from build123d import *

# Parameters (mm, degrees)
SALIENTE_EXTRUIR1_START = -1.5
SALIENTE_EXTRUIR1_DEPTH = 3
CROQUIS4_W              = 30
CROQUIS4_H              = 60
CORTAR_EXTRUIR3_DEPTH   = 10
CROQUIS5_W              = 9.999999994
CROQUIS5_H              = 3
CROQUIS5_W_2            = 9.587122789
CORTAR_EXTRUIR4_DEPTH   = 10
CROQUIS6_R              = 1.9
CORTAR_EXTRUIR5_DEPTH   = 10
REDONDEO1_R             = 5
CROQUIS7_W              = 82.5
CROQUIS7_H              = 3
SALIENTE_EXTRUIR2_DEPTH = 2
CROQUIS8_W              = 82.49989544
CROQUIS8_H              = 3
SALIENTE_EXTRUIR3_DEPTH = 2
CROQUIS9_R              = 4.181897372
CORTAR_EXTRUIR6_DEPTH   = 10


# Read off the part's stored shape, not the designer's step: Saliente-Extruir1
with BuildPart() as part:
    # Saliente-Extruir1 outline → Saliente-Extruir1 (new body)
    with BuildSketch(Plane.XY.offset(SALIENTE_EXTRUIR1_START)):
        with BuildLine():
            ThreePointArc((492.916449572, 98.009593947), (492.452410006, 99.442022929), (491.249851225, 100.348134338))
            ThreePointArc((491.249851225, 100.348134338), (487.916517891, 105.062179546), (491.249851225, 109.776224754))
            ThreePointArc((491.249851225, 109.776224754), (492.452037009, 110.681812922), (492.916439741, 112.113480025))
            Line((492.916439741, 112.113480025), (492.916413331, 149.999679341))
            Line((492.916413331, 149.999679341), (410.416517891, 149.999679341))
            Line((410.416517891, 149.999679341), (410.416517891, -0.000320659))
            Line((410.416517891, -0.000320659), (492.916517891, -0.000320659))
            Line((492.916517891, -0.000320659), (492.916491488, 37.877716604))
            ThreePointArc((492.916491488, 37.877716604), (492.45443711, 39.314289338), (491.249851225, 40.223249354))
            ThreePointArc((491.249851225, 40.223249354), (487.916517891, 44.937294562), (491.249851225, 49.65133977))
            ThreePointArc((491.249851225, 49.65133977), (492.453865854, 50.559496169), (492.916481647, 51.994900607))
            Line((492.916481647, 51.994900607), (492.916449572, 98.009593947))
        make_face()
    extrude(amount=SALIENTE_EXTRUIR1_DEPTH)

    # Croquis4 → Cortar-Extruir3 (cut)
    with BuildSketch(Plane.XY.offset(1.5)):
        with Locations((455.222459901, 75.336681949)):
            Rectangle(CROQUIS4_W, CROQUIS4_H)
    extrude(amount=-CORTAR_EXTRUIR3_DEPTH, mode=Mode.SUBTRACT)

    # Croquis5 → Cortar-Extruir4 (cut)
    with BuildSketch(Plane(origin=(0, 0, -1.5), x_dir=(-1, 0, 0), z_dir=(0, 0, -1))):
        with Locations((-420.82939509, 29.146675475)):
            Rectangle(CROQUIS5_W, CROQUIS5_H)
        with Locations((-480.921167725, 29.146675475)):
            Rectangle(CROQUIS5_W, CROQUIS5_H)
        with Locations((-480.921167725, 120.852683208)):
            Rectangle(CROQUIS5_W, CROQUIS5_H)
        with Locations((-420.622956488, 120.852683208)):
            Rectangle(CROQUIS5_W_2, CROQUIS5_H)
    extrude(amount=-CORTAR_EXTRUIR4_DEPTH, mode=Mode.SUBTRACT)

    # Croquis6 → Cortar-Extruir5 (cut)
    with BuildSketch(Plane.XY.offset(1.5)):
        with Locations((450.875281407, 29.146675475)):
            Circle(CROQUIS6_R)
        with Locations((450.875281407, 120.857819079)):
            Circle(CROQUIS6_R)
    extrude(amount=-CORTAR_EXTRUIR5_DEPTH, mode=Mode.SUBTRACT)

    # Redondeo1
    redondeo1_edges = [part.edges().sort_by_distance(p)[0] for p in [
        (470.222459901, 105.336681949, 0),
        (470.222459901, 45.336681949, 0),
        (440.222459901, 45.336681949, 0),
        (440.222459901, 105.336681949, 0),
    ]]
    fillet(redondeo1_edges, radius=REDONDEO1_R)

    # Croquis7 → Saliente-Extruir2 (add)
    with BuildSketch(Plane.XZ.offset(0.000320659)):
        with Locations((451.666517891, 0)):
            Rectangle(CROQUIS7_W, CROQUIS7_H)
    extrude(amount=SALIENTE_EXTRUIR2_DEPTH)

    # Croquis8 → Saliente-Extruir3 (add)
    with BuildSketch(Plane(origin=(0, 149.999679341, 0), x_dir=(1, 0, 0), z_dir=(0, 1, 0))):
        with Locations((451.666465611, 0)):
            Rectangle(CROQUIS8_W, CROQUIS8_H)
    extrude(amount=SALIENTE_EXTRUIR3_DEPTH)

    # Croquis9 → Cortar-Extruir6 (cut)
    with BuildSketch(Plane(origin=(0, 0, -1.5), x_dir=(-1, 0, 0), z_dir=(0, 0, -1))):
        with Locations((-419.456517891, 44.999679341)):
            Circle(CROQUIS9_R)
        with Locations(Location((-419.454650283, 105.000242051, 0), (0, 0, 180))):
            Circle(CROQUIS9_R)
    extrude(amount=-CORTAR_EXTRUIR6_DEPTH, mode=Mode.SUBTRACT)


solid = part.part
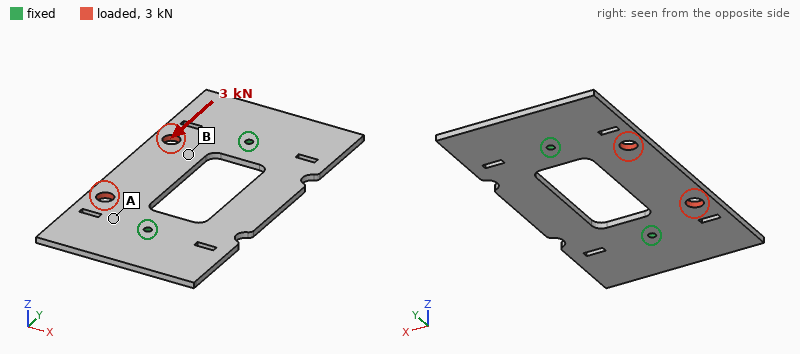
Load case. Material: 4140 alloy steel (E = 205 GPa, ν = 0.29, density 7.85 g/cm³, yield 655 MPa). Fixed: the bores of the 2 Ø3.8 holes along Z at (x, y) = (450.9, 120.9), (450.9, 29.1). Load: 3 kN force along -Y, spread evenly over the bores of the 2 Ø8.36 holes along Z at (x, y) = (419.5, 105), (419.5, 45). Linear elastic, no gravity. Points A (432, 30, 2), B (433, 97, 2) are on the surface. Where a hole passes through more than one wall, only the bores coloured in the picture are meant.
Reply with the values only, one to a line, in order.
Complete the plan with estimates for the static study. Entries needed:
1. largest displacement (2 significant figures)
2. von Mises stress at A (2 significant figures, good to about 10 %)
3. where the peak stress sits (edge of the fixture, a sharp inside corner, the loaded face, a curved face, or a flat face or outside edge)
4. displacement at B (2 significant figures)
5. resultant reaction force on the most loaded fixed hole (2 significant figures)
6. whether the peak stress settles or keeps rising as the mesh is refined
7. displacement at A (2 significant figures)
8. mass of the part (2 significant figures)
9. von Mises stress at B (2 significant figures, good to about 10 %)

17 µm
12 MPa
edge of the fixture
9.8 µm
1.8 kN
keeps rising
7.9 µm
250 g
30 MPa
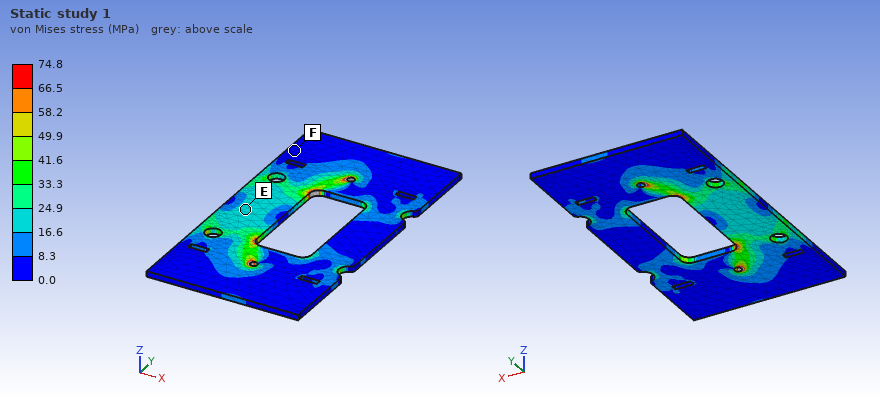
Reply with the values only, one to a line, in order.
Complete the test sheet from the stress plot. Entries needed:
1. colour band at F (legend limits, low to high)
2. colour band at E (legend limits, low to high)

0.0 to 8.3 MPa
16.6 to 24.9 MPa
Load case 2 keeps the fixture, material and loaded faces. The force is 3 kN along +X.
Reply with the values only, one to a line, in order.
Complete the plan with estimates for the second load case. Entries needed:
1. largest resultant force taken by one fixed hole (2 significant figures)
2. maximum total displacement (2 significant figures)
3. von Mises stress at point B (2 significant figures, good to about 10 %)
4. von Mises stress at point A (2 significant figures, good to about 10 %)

1.6 kN
7.4 µm
10 MPa
16 MPa
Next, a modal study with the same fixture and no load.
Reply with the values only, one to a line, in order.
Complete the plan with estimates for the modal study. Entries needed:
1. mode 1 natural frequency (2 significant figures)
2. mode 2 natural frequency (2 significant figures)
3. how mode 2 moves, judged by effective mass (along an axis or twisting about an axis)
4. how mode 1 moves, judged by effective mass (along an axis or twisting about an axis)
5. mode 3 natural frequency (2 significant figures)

840 Hz
1000 Hz
along Z
twisting about Y
1200 Hz
